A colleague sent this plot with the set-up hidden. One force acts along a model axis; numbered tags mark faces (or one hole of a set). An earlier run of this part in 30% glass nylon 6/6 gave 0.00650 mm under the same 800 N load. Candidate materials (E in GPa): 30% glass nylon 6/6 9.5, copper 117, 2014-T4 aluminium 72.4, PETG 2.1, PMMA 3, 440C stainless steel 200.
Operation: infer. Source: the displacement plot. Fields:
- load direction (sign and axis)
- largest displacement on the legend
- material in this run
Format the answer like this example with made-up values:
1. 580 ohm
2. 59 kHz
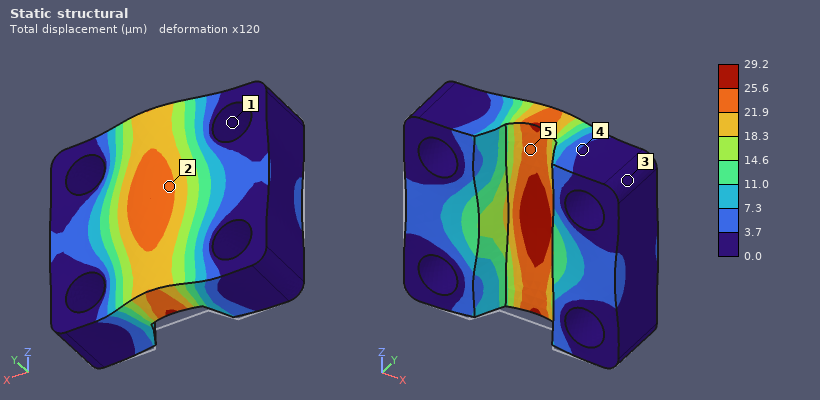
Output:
1. +Y
2. 29.2 µm
3. PETG
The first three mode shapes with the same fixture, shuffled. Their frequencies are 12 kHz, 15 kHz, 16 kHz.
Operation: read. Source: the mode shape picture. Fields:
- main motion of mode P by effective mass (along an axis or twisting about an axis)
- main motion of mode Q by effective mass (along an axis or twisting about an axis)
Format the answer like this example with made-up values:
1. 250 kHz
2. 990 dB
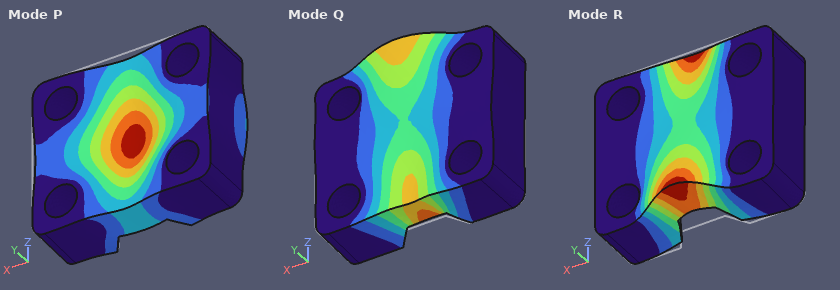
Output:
1. along Y
2. along Z
